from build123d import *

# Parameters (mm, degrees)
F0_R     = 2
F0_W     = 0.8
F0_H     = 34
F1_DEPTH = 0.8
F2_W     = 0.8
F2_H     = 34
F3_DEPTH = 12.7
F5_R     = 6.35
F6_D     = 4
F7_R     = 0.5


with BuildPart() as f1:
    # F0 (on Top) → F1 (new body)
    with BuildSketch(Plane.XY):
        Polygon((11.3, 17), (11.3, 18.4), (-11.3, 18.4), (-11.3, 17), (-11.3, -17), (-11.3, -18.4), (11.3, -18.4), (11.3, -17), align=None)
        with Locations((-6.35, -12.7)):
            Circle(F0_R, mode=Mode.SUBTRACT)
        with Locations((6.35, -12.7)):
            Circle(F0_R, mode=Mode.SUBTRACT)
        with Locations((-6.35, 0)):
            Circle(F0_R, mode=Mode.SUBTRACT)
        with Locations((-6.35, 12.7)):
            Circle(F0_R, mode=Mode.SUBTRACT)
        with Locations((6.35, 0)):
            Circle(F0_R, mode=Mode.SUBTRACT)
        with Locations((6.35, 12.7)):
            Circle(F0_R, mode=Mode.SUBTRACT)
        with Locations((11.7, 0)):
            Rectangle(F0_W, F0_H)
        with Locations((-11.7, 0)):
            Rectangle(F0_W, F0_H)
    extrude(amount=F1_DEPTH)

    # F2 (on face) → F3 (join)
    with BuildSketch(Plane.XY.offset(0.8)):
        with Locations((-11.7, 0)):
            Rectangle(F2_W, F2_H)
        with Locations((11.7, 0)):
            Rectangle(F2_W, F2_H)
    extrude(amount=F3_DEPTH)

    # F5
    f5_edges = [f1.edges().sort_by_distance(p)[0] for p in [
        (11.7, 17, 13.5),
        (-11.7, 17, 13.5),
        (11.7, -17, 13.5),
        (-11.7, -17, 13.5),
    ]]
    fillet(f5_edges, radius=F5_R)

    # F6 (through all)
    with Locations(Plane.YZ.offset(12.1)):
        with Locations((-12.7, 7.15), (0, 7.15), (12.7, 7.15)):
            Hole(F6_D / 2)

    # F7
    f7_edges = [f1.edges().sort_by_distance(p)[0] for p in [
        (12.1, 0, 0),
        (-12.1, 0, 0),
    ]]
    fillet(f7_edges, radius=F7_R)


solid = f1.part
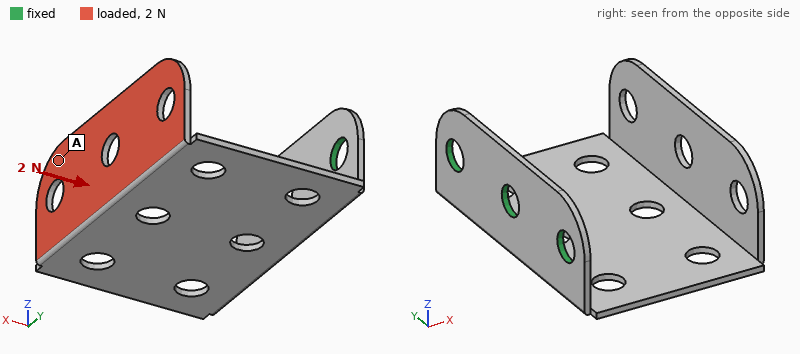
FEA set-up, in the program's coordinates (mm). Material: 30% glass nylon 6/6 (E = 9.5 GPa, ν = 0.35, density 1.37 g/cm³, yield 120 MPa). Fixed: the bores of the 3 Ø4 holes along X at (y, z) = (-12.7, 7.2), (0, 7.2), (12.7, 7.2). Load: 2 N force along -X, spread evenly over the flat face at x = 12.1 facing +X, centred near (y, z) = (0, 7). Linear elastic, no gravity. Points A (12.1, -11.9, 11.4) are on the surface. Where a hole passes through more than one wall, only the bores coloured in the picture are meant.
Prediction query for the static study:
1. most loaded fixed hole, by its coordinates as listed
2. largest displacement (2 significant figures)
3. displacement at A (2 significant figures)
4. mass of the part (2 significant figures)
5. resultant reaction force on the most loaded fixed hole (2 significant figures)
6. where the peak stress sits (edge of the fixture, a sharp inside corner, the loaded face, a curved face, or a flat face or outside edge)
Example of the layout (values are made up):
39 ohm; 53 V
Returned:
(0, 7.2); 0.48 mm; 0.44 mm; 1.7 g; 0.75 N; a curved face
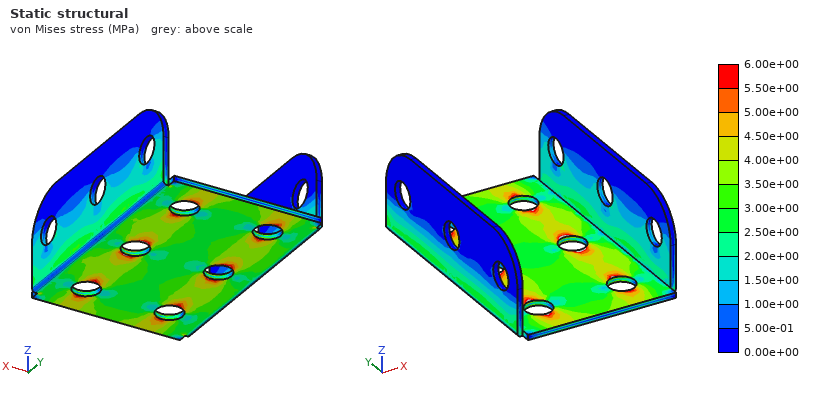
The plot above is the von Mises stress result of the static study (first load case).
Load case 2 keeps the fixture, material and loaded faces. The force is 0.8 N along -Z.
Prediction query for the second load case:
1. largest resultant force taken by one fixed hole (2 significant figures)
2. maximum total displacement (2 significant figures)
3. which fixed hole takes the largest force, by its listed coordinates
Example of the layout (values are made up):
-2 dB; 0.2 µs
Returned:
0.42 N; 0.51 mm; (0, 7.2)
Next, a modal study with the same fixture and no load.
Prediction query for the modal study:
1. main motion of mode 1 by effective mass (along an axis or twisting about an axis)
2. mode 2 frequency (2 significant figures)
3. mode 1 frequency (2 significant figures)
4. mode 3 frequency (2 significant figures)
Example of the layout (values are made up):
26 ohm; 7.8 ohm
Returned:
along Z; 560 Hz; 270 Hz; 1100 Hz
